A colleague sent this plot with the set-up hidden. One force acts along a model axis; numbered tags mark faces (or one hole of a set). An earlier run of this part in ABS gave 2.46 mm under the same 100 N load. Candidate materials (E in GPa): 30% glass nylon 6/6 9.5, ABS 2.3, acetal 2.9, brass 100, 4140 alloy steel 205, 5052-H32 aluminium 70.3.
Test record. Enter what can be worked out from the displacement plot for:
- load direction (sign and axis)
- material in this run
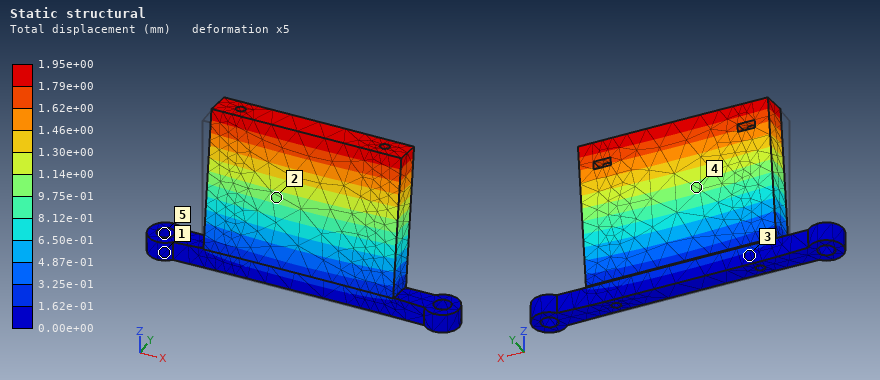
+Y
acetal
